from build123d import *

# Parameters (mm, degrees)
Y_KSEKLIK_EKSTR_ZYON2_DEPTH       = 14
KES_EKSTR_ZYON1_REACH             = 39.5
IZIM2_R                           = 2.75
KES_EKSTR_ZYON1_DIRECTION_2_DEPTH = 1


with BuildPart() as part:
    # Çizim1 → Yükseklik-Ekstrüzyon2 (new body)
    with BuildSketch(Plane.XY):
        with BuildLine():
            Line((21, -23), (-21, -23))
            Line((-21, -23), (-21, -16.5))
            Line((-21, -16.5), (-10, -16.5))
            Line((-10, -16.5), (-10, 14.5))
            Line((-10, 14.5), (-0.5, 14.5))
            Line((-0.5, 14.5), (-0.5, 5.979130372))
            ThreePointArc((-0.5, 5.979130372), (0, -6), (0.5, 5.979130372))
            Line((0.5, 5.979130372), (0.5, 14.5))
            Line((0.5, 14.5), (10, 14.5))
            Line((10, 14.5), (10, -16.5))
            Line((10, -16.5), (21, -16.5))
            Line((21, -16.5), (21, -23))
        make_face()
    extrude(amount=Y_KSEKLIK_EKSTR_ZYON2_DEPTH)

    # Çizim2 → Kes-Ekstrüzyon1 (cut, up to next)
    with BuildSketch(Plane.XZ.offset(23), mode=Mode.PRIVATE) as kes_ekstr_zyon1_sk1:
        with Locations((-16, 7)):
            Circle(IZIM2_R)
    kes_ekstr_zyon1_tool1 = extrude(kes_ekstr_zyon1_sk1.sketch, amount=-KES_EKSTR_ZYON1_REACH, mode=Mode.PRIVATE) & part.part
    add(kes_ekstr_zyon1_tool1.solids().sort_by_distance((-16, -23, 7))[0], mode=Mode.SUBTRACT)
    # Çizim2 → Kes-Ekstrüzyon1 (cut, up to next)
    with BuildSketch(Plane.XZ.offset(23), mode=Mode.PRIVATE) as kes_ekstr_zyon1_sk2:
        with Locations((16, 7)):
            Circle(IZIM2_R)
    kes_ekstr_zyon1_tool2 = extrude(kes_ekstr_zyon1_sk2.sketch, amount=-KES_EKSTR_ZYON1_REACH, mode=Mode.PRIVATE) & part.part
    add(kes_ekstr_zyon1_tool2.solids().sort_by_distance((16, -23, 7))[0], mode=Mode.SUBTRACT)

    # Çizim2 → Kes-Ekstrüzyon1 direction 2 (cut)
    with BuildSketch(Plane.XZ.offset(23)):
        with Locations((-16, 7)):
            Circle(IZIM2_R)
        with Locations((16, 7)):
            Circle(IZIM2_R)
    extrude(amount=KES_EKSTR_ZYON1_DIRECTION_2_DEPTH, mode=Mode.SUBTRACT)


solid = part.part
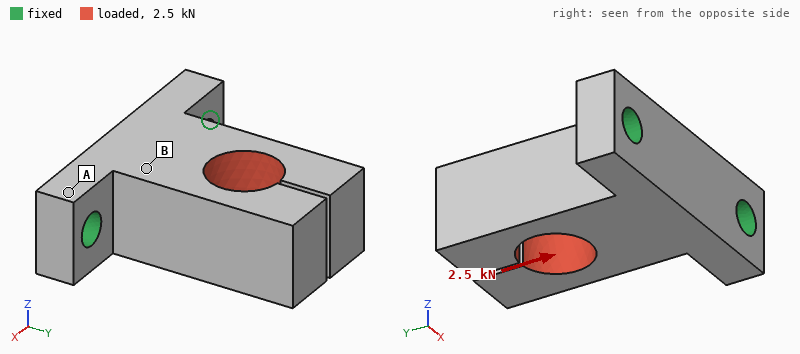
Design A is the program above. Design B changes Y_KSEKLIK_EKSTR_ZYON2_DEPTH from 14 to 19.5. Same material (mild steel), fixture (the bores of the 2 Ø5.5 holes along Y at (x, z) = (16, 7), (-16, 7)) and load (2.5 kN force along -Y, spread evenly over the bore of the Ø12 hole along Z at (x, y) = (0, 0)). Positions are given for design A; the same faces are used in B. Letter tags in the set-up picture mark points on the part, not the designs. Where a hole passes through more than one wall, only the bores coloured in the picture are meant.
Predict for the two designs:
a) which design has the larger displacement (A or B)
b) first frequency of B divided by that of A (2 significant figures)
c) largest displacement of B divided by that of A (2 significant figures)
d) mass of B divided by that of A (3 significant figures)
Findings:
A
1.0
0.80
1.40
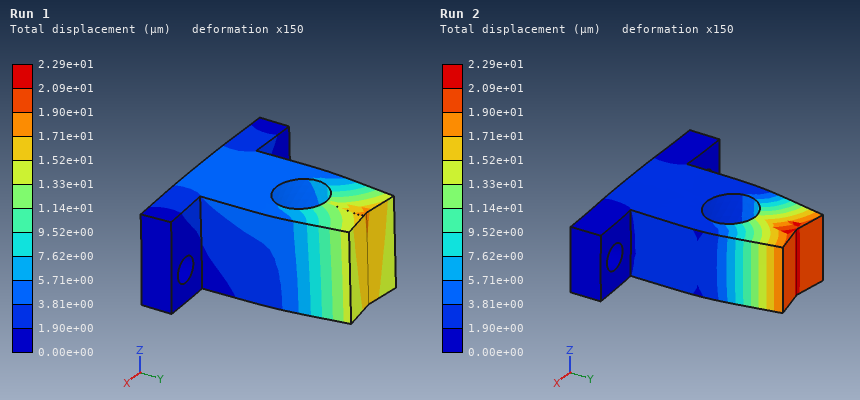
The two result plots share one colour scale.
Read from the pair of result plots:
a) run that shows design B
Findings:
Run 1
